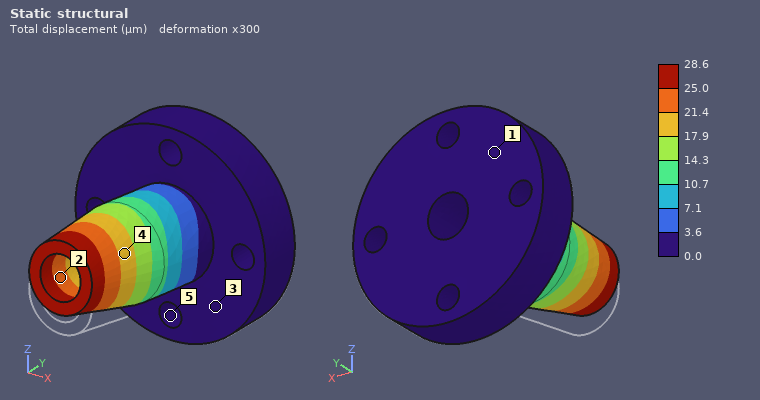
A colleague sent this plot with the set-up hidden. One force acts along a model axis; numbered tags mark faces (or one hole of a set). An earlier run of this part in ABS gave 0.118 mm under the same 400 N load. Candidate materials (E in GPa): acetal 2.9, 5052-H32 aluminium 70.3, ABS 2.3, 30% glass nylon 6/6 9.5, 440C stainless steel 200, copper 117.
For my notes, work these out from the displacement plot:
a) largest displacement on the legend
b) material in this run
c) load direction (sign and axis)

28.6 µm
30% glass nylon 6/6
+Z
